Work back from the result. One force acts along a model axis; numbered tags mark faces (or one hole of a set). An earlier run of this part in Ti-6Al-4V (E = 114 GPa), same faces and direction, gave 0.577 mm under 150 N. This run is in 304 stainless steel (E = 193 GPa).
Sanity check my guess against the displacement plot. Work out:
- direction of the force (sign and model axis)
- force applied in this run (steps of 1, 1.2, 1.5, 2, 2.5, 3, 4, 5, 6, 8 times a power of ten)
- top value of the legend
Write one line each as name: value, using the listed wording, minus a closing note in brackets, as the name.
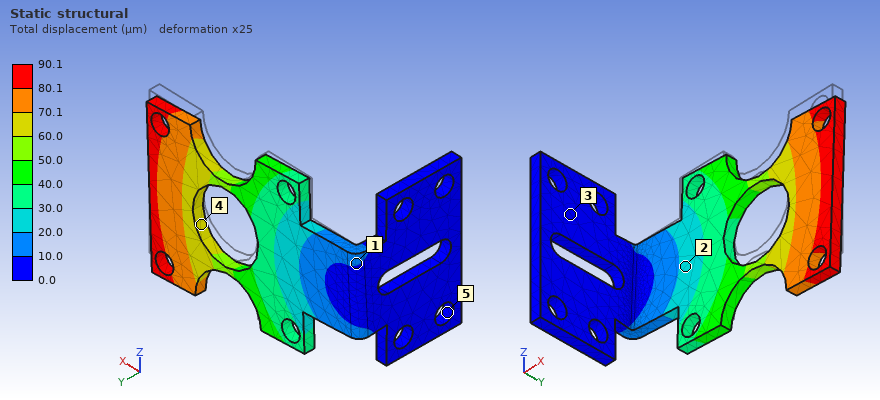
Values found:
direction of the force: -Z
force applied in this run: 40 N
top value of the legend: 90.1 µm
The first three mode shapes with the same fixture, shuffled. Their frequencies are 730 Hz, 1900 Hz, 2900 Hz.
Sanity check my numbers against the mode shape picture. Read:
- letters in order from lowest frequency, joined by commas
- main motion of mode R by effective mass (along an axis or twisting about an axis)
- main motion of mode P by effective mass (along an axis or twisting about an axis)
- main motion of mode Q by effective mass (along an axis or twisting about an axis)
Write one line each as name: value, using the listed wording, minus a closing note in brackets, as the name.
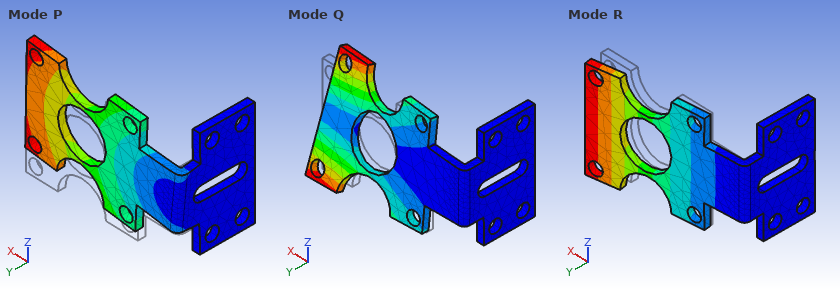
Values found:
letters in order from lowest frequency, joined by commas: R, P, Q
main motion of mode R by effective mass: along Y
main motion of mode P by effective mass: along Z
main motion of mode Q by effective mass: twisting about X
